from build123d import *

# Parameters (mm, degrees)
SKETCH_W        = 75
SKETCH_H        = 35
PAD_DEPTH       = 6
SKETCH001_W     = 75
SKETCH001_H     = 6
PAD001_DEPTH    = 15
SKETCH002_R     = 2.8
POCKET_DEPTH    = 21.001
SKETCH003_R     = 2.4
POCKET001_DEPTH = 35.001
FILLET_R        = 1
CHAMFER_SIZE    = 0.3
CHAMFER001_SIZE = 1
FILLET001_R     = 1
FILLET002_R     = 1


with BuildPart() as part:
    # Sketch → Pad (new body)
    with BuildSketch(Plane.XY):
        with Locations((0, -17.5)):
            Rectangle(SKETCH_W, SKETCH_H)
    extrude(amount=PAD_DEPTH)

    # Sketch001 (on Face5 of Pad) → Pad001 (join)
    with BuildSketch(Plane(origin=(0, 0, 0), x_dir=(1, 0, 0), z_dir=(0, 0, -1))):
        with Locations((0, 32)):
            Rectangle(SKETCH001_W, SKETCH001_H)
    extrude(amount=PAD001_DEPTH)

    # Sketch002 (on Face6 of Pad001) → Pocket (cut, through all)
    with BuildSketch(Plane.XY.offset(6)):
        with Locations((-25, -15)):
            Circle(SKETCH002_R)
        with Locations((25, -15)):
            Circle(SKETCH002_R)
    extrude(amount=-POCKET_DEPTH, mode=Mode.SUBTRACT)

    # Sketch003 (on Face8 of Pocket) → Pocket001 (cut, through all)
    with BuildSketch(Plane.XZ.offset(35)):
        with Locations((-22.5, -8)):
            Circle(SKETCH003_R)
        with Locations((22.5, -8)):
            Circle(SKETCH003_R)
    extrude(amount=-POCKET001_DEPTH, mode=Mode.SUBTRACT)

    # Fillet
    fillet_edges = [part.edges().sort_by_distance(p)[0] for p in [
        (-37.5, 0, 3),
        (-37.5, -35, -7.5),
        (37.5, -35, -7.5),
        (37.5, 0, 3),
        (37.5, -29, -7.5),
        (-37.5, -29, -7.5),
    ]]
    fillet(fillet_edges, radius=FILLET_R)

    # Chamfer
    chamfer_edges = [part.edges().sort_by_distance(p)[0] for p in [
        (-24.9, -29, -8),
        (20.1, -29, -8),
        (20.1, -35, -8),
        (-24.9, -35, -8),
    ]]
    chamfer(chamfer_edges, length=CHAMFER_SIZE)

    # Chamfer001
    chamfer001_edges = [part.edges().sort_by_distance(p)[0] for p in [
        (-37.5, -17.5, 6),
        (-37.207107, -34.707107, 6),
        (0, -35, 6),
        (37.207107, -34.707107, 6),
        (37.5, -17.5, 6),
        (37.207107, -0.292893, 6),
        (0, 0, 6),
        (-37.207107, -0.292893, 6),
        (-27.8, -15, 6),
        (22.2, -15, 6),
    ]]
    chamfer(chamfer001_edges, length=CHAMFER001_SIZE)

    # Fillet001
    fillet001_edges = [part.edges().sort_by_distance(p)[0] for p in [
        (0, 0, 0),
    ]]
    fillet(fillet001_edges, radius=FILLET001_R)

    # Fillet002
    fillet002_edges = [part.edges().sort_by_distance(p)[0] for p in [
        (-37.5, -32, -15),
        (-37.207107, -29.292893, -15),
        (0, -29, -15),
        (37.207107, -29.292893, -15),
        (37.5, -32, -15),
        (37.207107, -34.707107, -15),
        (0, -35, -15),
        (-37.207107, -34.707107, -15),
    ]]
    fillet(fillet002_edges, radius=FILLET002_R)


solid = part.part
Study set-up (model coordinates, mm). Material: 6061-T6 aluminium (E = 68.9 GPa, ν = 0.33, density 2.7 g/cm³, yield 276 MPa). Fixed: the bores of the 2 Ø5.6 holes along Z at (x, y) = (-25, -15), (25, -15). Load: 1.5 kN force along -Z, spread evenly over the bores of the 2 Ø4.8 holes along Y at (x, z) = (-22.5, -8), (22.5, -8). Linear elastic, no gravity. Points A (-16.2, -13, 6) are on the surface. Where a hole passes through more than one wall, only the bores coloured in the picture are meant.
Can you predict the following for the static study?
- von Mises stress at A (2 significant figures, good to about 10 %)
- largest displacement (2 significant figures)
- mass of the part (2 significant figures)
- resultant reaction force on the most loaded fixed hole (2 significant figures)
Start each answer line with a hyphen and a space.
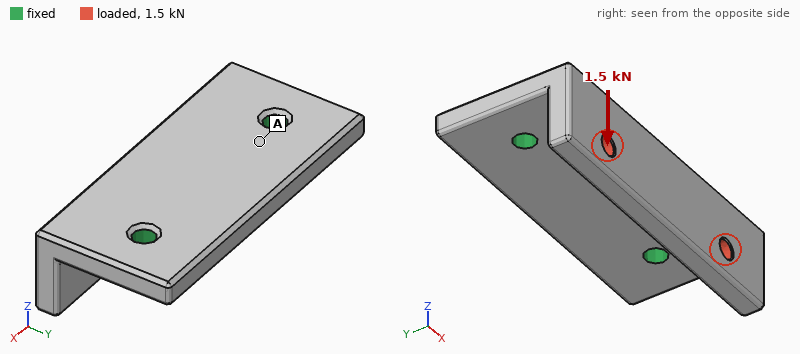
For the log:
- 19 MPa
- 74 µm
- 59 g
- 750 N
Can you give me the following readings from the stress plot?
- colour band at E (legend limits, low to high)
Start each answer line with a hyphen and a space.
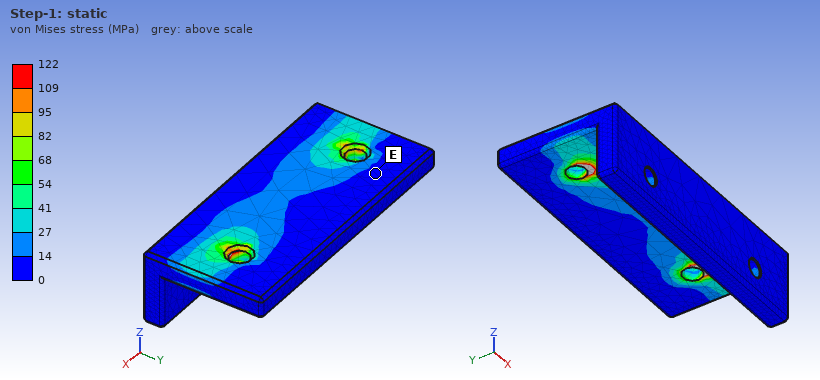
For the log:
- 0 to 14 MPa
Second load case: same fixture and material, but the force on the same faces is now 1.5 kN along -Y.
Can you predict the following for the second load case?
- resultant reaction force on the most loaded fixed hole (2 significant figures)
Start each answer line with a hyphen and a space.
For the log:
- 750 N
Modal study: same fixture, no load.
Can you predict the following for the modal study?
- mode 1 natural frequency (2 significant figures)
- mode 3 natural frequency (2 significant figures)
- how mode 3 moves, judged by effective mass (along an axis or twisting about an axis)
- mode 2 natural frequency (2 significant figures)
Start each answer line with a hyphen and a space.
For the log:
- 4600 Hz
- 11 kHz
- along Z
- 7000 Hz
